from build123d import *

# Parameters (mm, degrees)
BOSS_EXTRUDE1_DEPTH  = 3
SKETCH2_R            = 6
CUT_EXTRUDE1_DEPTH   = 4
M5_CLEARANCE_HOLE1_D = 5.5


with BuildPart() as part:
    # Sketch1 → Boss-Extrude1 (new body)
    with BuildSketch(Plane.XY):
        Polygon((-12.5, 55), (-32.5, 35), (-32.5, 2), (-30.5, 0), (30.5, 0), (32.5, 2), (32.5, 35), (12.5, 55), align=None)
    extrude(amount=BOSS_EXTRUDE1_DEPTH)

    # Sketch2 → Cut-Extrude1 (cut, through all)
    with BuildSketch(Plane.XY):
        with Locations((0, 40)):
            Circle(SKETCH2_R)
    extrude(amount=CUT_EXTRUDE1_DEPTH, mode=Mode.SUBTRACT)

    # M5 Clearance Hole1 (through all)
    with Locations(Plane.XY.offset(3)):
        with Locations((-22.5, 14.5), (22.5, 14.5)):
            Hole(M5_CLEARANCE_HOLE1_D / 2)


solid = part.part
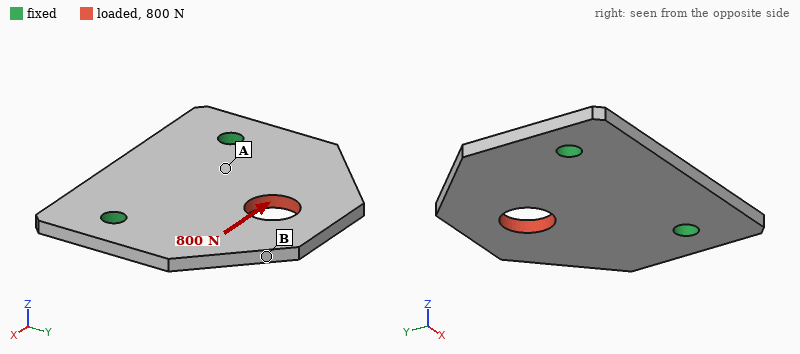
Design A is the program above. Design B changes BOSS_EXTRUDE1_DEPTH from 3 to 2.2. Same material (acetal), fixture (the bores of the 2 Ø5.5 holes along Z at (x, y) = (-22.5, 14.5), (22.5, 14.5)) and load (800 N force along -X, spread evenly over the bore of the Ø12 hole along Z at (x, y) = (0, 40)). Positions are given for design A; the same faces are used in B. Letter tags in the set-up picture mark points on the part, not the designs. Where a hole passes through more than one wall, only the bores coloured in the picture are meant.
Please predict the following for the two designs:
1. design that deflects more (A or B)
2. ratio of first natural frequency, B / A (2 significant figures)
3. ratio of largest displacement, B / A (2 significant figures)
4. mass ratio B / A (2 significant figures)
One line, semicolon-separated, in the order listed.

B; 0.75; 1.4; 0.73
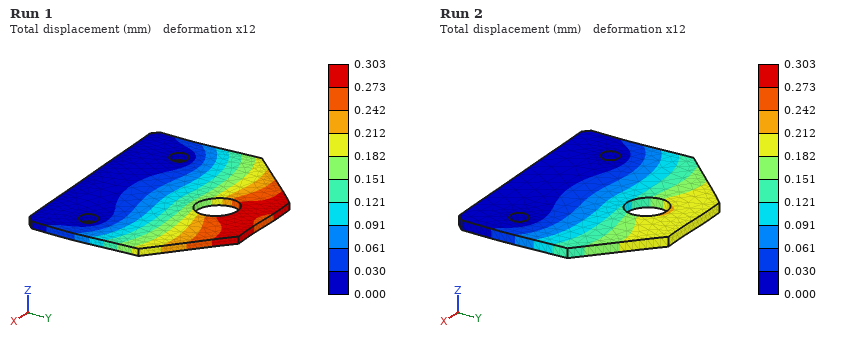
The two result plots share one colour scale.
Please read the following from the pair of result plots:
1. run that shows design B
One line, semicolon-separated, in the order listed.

Run 1
